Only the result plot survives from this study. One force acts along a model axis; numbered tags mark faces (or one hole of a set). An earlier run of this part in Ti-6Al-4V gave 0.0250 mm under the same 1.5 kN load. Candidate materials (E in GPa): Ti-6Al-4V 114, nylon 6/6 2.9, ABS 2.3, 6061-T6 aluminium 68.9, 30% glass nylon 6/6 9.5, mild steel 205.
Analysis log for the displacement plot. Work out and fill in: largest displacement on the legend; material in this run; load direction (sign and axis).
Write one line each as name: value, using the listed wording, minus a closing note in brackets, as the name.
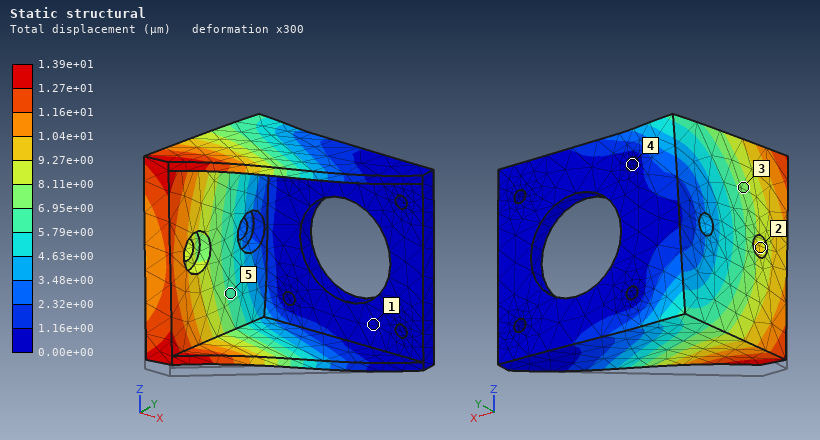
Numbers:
largest displacement on the legend: 1.39e+01 µm
material in this run: mild steel
load direction: +Z
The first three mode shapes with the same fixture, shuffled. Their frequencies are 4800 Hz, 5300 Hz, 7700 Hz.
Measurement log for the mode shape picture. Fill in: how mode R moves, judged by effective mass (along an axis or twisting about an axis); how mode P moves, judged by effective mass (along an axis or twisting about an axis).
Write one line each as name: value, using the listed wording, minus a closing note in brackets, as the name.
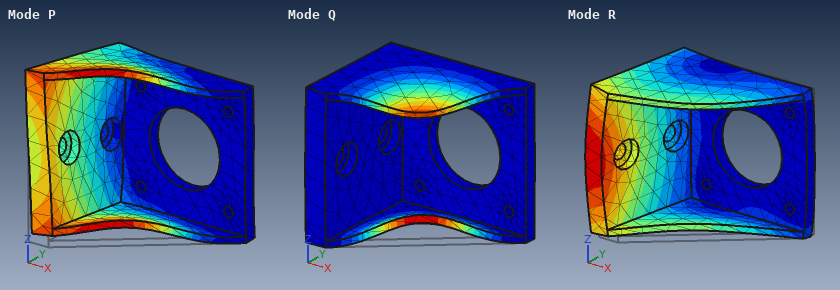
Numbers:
how mode R moves, judged by effective mass: along X
how mode P moves, judged by effective mass: along Z
